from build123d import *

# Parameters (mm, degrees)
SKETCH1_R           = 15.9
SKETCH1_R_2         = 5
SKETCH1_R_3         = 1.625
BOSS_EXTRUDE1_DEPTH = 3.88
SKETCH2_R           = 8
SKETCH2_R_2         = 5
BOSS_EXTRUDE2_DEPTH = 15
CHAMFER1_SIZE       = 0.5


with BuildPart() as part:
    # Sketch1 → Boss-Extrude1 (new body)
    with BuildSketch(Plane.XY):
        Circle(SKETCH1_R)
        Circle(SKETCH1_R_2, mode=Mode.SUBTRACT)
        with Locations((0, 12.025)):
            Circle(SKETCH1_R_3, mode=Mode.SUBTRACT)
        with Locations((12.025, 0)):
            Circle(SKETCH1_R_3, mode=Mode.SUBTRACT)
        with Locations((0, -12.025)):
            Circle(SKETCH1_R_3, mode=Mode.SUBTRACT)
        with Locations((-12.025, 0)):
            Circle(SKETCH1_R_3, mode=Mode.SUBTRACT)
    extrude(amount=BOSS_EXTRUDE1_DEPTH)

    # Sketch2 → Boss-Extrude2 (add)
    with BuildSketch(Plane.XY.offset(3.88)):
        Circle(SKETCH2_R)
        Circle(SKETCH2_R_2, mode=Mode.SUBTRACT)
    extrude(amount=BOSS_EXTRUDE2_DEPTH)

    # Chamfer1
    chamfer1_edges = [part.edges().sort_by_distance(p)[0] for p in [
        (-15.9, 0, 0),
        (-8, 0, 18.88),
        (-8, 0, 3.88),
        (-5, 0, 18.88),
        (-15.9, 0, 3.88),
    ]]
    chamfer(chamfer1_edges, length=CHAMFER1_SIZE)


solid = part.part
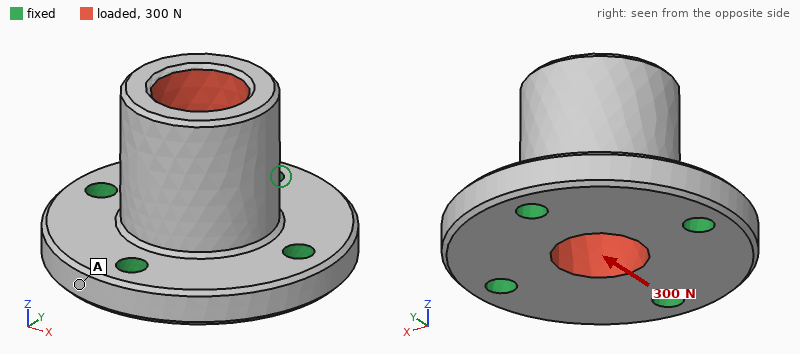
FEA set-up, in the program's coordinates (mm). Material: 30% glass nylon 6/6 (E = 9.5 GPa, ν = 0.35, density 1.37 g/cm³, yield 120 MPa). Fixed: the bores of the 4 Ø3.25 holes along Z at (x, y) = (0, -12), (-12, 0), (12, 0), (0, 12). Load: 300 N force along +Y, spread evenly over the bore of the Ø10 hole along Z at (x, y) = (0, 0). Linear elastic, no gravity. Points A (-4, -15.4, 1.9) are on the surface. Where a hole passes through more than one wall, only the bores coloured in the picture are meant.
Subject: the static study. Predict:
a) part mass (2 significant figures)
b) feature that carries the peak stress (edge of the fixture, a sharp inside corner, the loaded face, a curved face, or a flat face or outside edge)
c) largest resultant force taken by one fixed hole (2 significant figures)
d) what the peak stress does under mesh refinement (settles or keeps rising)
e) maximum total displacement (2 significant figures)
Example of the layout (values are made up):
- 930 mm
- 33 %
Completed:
- 6.1 g
- edge of the fixture
- 140 N
- keeps rising
- 22 µm
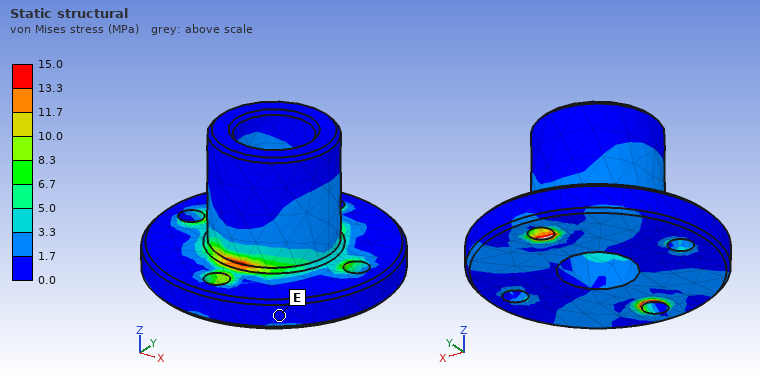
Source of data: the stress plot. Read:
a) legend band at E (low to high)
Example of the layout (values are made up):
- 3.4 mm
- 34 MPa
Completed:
- 0.0 to 1.7 MPa
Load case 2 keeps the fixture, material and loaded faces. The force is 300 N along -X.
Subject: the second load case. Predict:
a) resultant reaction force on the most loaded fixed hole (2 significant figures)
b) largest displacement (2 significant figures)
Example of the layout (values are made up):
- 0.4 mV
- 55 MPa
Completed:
- 140 N
- 22 µm
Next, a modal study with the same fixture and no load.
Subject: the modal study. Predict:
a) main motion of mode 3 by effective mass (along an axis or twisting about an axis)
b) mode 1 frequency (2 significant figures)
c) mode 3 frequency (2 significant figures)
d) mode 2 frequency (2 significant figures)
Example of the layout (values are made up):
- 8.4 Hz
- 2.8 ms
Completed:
- along Z
- 12 kHz
- 19 kHz
- 12 kHz
